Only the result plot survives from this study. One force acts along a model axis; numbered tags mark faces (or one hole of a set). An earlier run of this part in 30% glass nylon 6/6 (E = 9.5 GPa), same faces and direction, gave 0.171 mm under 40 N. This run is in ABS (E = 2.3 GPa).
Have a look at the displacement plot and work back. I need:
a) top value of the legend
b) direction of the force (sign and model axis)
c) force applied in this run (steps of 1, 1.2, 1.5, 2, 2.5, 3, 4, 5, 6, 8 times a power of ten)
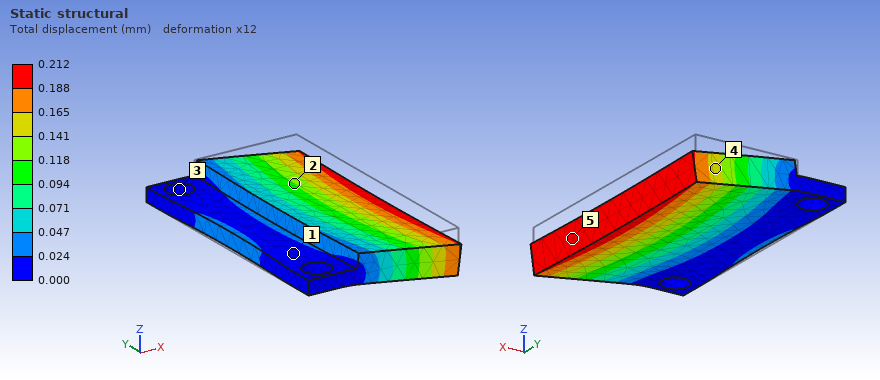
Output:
0.212 mm
-Z
12 N
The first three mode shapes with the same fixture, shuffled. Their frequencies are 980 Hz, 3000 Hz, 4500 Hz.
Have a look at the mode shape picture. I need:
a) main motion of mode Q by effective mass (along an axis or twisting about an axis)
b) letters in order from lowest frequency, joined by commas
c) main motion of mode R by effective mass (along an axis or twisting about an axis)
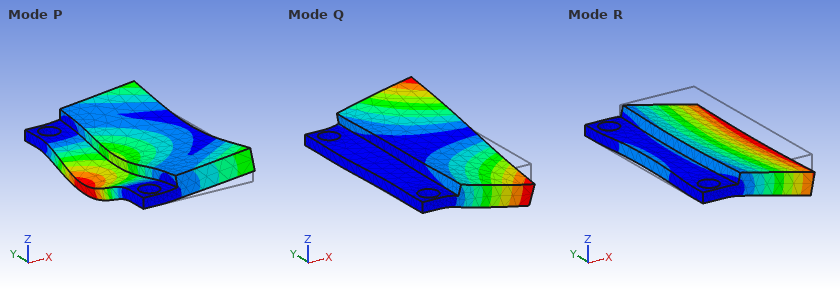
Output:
twisting about X
R, Q, P
along Z
